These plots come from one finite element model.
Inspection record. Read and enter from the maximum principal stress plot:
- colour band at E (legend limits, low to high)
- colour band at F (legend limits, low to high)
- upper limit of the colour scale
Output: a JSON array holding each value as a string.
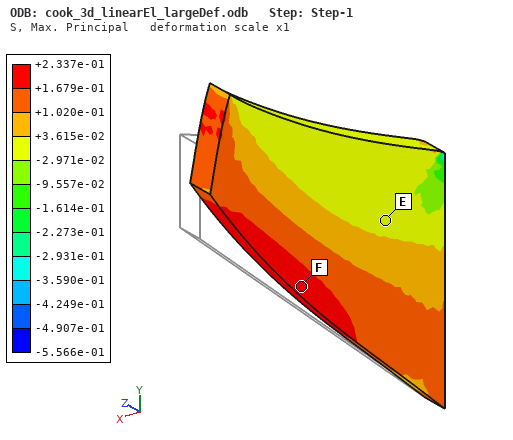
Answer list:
["-2.971e-02 to +3.615e-02", "+1.679e-01 to +2.337e-01", "+2.337e-01"]
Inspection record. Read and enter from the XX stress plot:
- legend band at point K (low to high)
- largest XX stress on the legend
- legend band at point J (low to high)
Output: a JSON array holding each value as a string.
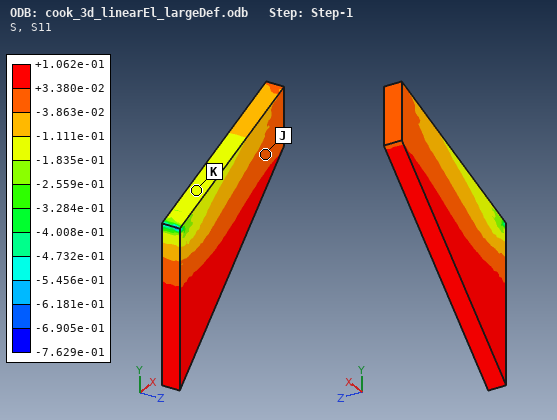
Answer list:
["-1.835e-01 to -1.111e-01", "+1.062e-01", "-3.863e-02 to +3.380e-02"]
